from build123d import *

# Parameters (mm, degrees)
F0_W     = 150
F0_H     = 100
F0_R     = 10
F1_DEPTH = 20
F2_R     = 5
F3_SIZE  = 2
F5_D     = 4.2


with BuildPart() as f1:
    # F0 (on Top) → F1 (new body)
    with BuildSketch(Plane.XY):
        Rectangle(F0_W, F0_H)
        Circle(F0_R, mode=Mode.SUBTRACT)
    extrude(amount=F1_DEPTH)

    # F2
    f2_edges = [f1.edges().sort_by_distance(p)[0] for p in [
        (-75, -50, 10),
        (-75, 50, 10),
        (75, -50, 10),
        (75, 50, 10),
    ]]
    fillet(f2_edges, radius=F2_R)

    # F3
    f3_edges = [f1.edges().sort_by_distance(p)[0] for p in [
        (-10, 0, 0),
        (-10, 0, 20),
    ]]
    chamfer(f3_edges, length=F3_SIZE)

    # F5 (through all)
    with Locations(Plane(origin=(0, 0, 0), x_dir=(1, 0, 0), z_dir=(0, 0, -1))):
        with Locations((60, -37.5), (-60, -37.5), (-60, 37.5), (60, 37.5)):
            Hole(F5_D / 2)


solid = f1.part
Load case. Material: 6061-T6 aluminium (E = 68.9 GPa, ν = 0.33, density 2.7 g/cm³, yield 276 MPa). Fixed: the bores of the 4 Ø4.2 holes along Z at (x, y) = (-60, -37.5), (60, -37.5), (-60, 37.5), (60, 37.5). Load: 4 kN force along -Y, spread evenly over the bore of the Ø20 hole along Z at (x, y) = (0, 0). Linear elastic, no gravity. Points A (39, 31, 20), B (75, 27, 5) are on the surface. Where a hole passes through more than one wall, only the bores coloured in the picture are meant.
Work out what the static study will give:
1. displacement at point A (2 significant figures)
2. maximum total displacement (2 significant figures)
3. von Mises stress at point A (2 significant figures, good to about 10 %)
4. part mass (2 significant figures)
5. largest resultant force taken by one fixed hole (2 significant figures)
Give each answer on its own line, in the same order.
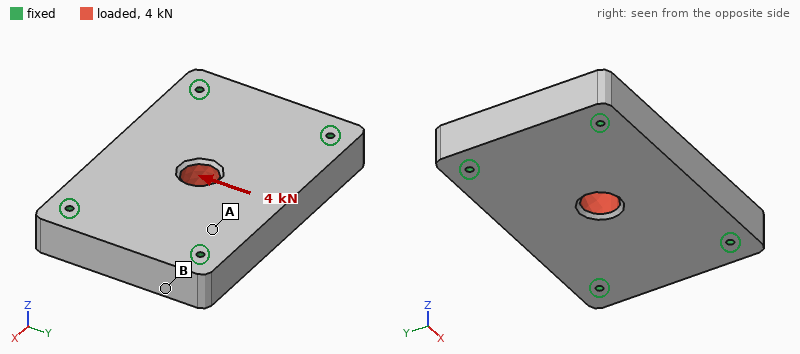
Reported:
1.4 µm
3.7 µm
2.0 MPa
790 g
1.2 kN
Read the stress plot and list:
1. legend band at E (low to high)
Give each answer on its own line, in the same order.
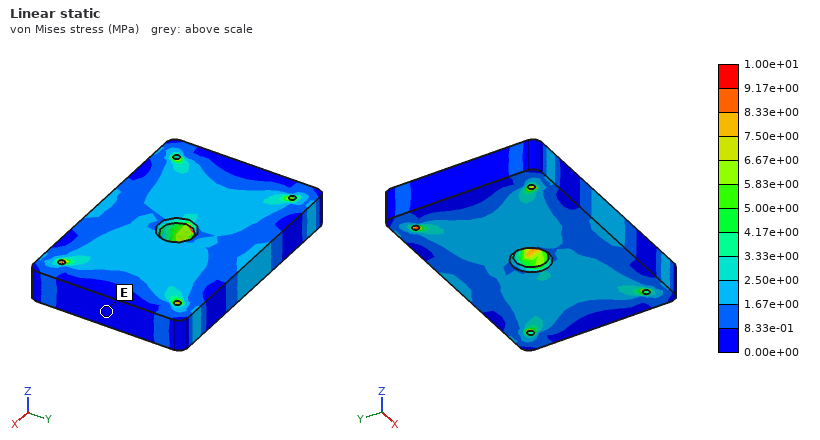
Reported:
0.00e+00 to 8.33e-01 MPa
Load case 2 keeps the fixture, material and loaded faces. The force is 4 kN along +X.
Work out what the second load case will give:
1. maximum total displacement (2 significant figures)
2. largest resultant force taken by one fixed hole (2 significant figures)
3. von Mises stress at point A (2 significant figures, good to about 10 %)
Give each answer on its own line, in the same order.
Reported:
2.2 µm
1.0 kN
1.7 MPa
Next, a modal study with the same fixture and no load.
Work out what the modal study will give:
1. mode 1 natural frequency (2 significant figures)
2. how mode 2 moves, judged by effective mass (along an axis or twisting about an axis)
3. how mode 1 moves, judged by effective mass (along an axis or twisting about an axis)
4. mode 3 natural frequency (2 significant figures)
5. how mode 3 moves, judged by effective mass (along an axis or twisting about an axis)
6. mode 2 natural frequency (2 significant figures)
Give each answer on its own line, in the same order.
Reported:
4600 Hz
twisting about X
along Z
10 kHz
along Y
6800 Hz
